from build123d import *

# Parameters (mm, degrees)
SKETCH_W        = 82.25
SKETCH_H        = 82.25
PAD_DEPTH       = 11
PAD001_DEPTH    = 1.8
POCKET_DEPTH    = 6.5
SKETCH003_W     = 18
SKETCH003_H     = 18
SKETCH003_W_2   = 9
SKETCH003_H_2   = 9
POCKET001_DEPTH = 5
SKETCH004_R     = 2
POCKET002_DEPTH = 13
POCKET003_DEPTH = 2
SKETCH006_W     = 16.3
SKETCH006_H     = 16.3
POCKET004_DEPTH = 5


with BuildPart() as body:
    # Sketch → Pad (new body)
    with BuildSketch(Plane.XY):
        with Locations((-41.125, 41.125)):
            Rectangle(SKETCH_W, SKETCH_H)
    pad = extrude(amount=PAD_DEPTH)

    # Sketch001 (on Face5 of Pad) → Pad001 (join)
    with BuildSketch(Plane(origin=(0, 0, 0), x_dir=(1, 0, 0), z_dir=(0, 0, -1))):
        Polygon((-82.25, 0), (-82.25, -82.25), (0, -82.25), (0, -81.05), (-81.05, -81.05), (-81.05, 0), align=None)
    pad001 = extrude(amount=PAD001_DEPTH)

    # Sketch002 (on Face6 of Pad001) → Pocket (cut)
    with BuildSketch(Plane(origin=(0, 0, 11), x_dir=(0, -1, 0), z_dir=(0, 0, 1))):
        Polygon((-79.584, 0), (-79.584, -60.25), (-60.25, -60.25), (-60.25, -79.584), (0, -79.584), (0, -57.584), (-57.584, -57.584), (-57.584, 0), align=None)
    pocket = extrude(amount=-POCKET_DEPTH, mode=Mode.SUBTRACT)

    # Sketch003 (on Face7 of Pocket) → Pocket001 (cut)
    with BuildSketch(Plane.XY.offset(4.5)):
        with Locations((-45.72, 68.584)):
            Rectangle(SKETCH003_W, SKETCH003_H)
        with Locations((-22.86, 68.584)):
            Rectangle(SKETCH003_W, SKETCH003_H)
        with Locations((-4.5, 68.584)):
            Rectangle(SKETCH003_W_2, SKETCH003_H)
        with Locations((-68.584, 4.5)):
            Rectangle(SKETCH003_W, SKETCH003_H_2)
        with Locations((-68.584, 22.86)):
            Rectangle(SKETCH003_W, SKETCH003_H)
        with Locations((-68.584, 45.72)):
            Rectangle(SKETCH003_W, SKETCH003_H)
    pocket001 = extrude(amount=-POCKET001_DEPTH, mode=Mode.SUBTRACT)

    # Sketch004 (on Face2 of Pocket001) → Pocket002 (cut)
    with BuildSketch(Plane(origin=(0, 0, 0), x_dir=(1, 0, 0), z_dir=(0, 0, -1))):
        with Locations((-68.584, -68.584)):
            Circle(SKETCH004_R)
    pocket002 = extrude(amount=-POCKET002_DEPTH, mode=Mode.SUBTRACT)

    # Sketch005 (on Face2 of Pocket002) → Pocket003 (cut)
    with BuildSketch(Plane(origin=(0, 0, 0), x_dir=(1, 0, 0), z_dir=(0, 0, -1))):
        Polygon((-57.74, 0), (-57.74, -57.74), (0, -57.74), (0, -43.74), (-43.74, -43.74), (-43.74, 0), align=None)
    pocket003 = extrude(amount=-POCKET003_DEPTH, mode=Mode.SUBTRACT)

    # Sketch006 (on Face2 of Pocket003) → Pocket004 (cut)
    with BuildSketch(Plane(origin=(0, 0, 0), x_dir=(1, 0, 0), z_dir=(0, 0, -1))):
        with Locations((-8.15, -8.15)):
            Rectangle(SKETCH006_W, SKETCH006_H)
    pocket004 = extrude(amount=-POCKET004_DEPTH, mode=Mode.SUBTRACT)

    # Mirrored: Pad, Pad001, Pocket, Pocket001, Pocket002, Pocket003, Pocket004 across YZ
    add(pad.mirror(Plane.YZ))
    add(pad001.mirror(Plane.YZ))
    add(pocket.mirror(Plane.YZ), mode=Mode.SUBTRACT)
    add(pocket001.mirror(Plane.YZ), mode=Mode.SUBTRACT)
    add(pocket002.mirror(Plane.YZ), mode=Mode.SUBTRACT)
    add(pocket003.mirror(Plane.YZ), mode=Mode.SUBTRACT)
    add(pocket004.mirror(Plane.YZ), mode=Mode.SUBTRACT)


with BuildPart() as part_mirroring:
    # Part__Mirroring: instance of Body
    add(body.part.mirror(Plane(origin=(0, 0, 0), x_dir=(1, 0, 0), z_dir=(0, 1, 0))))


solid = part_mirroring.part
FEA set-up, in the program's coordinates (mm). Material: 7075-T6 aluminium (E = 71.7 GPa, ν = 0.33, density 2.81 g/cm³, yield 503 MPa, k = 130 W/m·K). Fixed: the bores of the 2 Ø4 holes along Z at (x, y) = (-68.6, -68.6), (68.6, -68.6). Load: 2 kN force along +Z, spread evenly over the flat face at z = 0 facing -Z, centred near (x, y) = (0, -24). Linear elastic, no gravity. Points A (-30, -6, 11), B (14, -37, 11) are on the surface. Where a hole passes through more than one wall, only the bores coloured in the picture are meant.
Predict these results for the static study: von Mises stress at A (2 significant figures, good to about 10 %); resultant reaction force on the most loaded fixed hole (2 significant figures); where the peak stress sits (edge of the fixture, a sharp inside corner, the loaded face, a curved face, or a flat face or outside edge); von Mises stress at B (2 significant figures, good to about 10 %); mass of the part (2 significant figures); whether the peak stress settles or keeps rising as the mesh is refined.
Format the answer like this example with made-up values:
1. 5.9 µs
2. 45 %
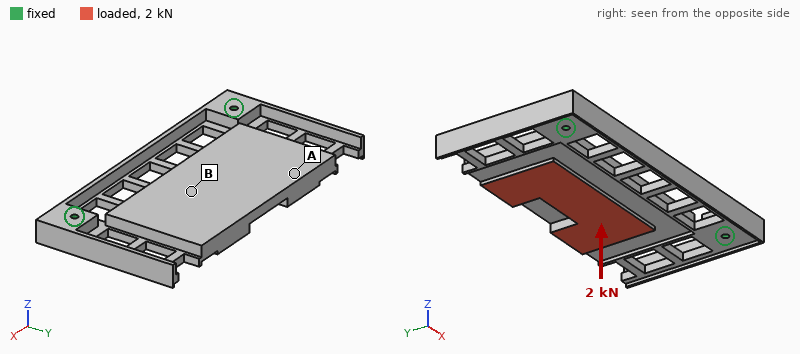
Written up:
1. 27 MPa
2. 1.2 kN
3. a sharp inside corner
4. 49 MPa
5. 260 g
6. keeps rising
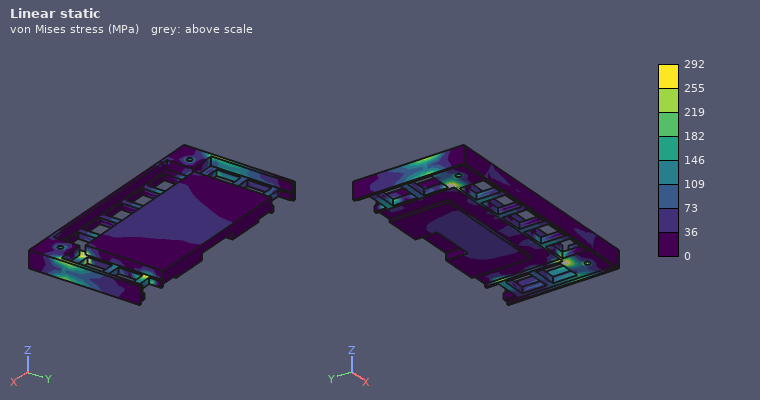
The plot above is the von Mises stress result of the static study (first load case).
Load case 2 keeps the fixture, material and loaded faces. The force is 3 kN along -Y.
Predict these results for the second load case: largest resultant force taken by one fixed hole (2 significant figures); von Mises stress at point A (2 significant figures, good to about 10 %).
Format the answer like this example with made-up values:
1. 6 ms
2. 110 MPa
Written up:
1. 1.6 kN
2. 7.3 MPa
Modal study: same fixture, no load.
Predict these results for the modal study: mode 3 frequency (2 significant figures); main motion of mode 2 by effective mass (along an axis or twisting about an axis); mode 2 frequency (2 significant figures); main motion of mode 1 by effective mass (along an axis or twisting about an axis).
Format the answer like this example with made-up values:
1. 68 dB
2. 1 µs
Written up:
1. 2400 Hz
2. twisting about Y
3. 1900 Hz
4. along Z
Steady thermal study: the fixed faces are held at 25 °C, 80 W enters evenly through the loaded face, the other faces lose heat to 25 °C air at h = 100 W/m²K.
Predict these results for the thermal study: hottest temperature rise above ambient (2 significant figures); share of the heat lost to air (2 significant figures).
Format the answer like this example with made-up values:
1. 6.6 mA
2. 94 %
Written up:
1. 36 K
2. 74 %
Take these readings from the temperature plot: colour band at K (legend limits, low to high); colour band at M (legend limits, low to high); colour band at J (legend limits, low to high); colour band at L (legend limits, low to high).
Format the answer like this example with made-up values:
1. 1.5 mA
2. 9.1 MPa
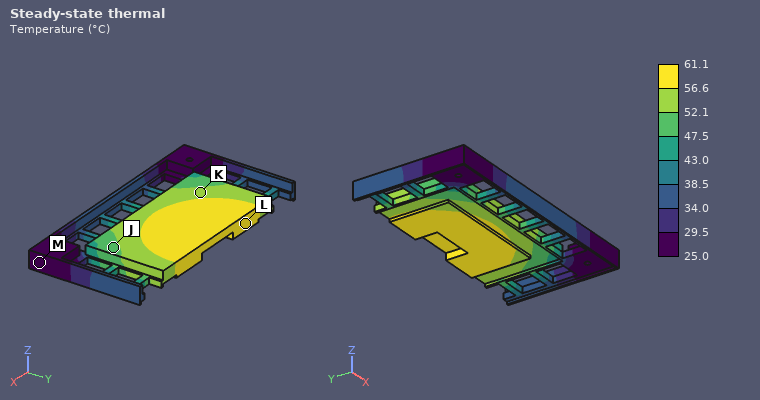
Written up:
1. 52.1 to 56.6 °C
2. 25.0 to 29.5 °C
3. 47.5 to 52.1 °C
4. 56.6 to 61.1 °C
